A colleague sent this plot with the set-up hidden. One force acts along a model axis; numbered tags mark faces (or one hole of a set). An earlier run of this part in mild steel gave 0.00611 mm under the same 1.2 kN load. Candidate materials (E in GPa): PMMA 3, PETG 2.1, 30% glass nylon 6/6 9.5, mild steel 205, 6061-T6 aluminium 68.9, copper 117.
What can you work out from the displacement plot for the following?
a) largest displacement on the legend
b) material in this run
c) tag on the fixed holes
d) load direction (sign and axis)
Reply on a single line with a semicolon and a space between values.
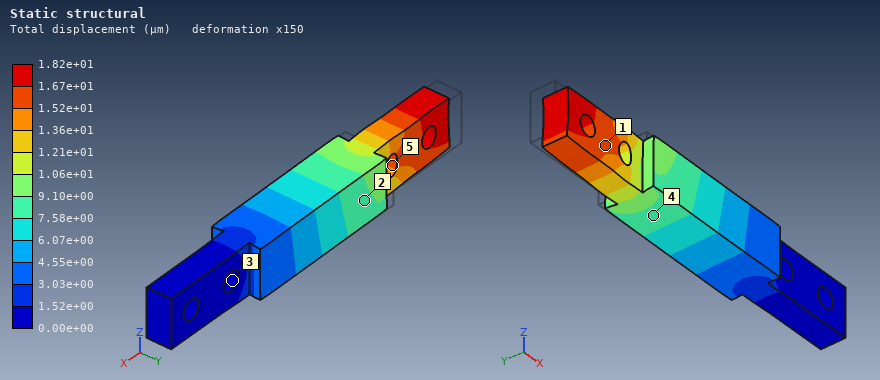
1.82e+01 µm; 6061-T6 aluminium; 3; +X
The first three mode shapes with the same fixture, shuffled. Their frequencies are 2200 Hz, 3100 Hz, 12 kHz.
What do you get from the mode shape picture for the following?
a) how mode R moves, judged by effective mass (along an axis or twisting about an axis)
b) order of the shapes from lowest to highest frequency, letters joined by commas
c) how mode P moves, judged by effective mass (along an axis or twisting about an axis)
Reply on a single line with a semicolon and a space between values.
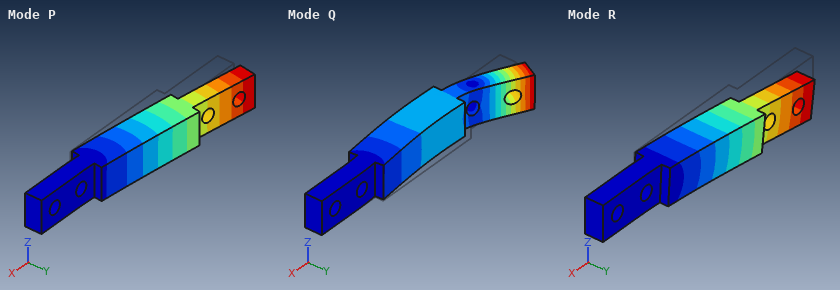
along Z; P, R, Q; along Y
